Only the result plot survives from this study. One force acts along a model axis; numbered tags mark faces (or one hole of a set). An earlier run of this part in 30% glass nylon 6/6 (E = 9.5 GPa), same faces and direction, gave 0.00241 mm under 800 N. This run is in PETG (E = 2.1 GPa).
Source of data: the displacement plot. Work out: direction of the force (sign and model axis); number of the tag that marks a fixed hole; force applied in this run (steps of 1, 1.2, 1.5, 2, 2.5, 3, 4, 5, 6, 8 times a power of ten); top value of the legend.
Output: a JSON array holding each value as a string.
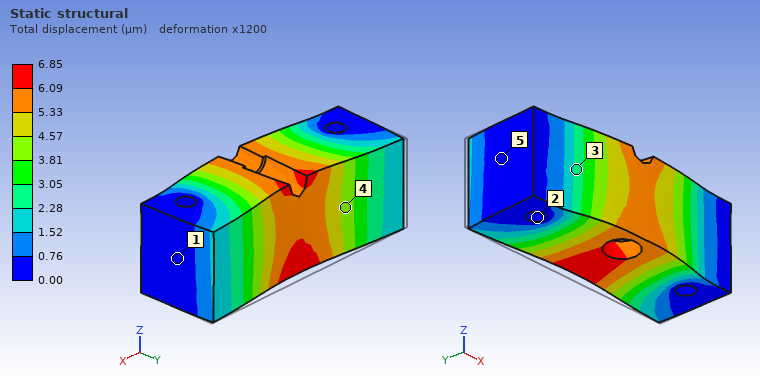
["-Y", "2", "500 N", "6.85 µm"]
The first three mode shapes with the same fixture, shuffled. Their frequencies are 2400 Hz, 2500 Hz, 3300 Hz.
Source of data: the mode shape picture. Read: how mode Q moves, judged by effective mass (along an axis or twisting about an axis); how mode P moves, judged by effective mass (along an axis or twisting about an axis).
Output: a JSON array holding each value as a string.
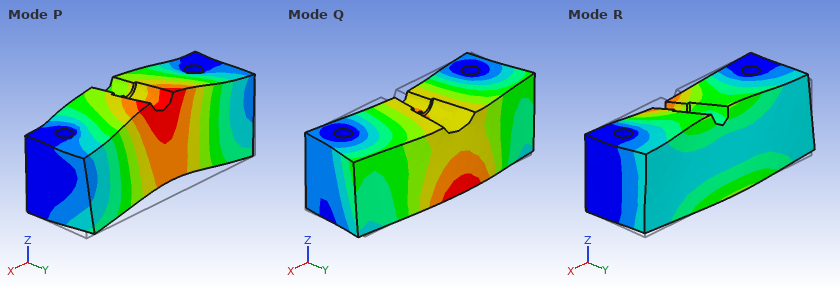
["along Y", "along Z"]
